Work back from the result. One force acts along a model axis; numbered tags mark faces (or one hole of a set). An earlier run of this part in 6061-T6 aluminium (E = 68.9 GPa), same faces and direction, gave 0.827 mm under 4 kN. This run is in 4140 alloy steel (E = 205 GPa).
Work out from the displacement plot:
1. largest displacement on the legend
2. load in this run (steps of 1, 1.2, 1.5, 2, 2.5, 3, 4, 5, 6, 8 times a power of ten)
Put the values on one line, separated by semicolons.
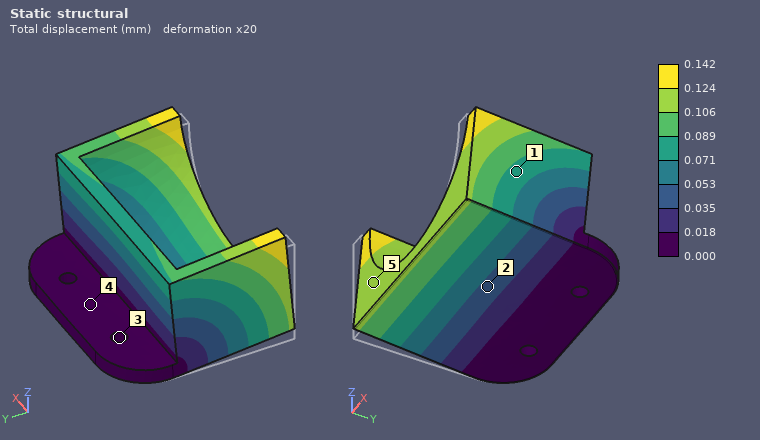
0.142 mm; 2 kN
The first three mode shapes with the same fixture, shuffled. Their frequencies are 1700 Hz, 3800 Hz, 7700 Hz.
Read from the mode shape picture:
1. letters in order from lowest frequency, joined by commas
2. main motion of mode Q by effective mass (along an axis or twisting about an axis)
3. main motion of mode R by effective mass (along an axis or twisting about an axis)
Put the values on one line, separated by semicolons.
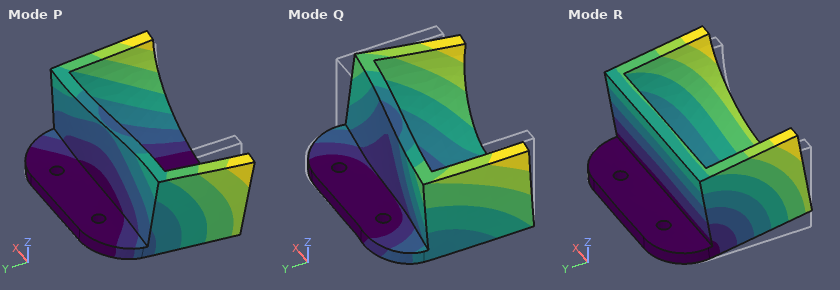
R, P, Q; along X; along Z
